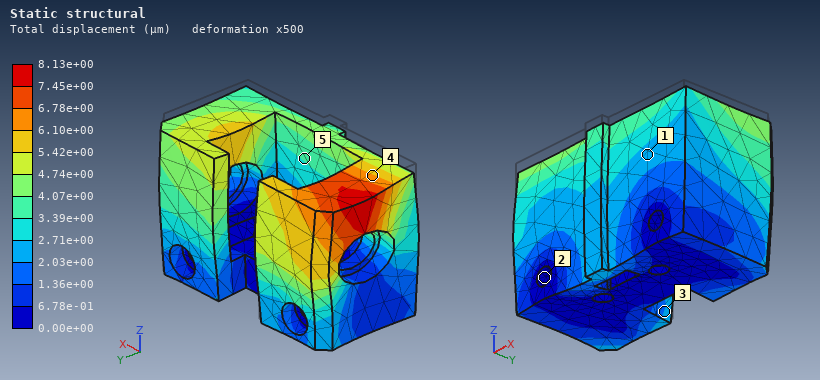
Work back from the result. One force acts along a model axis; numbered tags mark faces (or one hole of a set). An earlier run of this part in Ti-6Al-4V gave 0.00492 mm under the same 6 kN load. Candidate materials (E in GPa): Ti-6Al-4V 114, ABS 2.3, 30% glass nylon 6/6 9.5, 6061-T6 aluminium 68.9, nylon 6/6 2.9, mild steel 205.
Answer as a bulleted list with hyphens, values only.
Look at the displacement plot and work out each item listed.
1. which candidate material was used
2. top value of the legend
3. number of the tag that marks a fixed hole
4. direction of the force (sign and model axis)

- 6061-T6 aluminium
- 8.13e+00 µm
- 2
- -Z
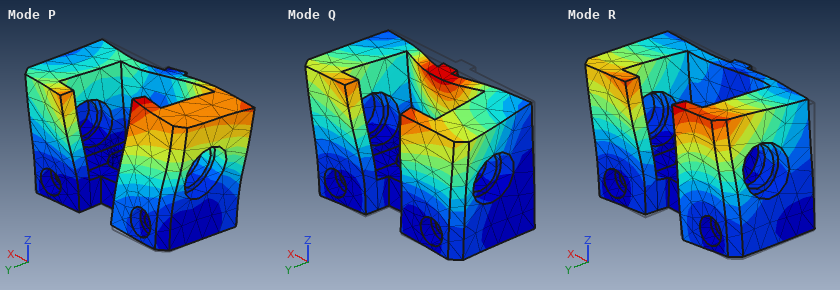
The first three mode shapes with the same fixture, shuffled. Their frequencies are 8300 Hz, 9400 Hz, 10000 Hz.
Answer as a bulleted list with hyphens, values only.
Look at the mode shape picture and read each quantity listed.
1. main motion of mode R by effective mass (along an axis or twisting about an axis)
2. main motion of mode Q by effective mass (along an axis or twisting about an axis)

- along X
- along Y
